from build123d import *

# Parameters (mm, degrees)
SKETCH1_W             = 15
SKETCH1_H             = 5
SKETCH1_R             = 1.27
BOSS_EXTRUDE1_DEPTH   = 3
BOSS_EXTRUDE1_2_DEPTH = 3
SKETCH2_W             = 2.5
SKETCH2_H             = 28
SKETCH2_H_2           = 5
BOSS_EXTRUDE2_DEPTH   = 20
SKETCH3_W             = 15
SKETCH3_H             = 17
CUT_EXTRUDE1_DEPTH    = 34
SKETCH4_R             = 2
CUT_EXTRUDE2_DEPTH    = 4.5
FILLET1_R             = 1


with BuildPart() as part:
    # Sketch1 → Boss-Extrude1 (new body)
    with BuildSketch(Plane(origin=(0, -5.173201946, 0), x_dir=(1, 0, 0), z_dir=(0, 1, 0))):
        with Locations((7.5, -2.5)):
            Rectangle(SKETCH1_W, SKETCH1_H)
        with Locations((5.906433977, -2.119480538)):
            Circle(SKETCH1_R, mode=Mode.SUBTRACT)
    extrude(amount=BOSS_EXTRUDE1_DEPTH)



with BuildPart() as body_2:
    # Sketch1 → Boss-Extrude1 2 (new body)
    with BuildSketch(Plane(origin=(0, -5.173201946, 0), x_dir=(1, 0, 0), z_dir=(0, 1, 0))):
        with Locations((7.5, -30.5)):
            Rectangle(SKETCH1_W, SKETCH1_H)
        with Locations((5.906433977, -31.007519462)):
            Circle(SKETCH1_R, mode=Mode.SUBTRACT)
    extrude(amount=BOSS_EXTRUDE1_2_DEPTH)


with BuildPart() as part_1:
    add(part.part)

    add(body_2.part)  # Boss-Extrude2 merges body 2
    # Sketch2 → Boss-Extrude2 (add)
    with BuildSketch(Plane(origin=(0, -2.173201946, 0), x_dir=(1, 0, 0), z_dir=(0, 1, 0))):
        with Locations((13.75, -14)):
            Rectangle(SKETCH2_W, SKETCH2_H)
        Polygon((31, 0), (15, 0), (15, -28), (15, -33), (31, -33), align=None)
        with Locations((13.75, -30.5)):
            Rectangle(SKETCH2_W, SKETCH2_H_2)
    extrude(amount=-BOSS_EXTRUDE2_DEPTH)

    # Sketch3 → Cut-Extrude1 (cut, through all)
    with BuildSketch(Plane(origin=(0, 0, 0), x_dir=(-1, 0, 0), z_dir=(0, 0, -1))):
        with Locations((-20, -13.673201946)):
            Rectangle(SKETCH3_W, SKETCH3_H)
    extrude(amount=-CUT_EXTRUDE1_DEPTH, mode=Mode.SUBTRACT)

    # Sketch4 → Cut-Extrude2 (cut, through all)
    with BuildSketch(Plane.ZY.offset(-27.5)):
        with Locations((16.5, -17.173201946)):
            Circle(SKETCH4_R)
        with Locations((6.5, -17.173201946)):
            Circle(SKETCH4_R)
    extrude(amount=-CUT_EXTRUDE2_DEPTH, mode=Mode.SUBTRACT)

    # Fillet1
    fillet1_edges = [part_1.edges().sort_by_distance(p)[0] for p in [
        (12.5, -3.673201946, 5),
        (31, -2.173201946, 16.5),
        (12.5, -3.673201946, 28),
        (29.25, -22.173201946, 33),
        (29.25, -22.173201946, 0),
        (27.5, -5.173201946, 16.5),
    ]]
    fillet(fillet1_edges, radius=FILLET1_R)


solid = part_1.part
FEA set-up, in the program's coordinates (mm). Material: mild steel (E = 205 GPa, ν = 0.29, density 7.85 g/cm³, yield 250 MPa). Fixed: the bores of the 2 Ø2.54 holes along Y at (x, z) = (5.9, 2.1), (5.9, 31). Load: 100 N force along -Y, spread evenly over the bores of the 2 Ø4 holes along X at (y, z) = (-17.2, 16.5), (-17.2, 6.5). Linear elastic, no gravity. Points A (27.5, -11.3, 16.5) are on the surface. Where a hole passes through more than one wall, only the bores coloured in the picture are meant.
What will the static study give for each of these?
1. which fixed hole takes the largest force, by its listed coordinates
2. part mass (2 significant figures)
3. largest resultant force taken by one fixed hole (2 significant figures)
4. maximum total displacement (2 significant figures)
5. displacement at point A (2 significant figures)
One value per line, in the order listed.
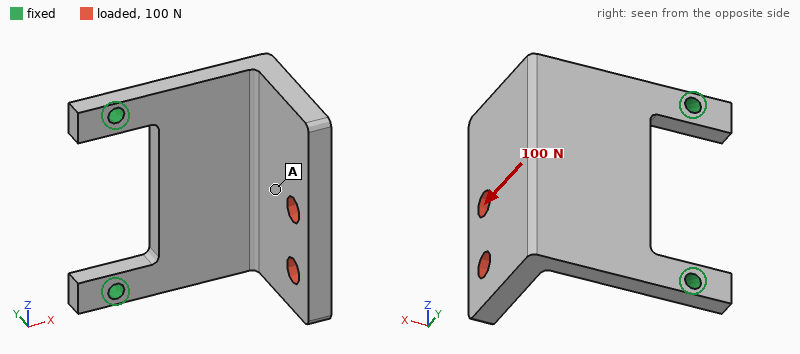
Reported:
(5.9, 2.1)
32 g
66 N
0.11 mm
0.071 mm
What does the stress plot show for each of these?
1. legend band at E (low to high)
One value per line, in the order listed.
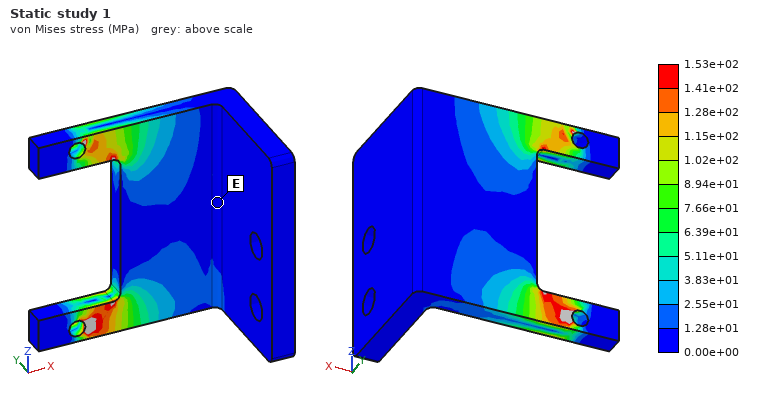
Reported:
0.00e+00 to 1.28e+01 MPa
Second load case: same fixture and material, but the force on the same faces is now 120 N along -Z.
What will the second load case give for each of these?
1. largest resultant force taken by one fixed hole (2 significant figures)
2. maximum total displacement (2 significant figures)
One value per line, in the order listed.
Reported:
110 N
24 µm
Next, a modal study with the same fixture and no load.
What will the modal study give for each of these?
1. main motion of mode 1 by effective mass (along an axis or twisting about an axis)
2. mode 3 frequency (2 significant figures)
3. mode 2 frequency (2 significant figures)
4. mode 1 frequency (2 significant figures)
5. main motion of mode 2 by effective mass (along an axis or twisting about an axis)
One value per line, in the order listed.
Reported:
along Y
5300 Hz
3300 Hz
1100 Hz
along Z
